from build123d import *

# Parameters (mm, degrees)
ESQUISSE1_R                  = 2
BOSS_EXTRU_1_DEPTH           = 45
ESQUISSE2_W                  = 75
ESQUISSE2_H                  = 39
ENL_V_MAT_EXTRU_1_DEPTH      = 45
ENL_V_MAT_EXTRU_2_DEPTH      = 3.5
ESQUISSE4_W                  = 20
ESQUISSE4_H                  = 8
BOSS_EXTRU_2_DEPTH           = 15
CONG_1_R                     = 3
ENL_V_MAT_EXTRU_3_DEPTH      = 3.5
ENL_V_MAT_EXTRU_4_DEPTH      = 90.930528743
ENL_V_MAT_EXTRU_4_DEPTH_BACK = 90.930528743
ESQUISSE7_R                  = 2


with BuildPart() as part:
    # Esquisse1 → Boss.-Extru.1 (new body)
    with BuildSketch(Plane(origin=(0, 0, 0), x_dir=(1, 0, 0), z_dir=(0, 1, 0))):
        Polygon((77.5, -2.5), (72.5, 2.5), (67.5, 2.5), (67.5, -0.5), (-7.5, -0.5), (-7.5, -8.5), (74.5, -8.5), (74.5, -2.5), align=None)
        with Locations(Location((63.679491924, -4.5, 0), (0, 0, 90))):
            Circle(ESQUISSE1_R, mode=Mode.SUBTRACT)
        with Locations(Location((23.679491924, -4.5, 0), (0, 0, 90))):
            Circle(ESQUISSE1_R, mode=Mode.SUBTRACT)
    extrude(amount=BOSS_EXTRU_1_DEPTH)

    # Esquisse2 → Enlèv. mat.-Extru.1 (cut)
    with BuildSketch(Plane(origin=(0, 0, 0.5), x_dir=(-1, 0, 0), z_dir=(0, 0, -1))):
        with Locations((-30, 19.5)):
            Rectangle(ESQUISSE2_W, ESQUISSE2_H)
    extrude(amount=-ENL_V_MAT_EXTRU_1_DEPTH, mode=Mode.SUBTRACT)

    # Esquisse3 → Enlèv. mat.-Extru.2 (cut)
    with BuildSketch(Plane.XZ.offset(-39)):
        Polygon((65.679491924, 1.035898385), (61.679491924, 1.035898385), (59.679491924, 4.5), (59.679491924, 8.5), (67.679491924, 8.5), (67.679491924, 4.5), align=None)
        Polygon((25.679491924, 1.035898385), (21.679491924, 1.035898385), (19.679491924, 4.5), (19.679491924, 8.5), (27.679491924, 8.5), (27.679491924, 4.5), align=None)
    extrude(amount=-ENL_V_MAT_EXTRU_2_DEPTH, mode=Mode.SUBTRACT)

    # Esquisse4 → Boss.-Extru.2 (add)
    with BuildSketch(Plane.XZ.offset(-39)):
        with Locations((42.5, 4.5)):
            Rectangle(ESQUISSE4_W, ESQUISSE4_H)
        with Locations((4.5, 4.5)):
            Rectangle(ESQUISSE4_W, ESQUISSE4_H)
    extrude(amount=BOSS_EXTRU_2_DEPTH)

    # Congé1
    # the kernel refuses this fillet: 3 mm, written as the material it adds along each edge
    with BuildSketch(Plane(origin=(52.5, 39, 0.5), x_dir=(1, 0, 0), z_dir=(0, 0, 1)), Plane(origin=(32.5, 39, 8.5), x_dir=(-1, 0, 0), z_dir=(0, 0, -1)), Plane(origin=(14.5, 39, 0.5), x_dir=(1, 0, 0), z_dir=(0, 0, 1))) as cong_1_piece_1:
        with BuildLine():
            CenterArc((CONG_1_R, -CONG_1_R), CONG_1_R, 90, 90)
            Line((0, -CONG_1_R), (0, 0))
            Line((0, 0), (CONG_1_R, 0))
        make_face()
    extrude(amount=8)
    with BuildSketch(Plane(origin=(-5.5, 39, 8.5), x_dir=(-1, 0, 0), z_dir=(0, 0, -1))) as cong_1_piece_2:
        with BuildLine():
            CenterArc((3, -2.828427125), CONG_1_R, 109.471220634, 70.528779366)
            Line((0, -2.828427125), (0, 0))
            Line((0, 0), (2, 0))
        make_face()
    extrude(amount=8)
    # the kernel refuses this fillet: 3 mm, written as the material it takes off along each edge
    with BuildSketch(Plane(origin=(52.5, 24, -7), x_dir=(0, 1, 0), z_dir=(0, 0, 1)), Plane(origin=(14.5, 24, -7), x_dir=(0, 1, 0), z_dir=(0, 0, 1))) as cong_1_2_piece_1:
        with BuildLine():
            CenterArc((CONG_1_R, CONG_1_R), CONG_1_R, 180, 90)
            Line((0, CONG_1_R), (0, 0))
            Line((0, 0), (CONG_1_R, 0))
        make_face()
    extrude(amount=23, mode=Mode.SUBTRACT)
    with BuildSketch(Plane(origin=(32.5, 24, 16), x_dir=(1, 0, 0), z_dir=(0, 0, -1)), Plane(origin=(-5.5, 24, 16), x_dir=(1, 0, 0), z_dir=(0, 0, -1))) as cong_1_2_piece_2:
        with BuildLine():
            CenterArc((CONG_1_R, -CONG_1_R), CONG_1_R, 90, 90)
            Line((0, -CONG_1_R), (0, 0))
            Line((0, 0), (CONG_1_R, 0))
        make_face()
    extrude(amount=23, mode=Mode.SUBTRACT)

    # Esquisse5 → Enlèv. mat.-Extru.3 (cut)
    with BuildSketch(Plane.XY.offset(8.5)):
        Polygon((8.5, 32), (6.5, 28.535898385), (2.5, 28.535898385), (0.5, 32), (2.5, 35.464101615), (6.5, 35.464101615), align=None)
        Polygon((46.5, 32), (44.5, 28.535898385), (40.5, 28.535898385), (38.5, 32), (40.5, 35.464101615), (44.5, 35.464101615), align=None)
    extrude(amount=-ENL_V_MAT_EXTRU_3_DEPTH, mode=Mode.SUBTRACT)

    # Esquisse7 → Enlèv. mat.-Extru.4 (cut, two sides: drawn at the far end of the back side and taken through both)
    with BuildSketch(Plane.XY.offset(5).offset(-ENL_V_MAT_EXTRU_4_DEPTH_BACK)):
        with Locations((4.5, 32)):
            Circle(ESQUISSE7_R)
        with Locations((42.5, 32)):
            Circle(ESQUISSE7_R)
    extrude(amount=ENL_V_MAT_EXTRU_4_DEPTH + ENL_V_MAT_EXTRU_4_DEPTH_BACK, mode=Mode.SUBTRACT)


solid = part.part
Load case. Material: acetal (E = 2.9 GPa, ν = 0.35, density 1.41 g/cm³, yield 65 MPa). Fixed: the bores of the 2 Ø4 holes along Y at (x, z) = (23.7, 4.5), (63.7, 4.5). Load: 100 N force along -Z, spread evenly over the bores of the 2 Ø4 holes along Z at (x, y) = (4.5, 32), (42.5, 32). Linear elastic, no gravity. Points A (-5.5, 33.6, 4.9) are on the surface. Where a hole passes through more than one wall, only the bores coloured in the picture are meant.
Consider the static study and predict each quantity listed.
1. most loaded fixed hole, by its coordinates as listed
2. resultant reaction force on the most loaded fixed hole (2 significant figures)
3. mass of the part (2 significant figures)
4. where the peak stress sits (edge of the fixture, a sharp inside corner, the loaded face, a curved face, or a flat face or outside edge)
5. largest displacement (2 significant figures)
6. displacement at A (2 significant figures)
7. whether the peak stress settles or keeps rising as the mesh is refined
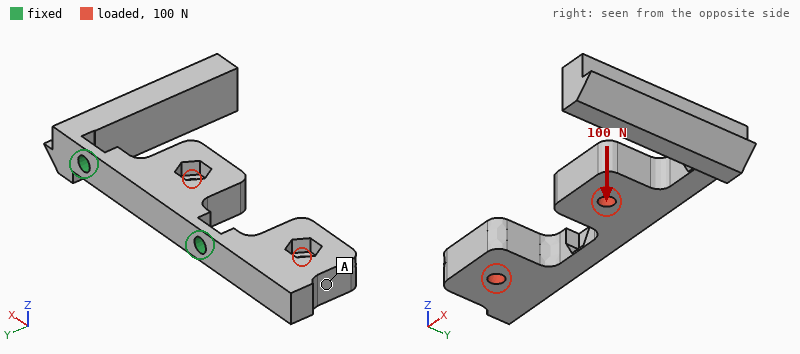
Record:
(23.7, 4.5)
81 N
16 g
edge of the fixture
1.1 mm
0.81 mm
keeps rising
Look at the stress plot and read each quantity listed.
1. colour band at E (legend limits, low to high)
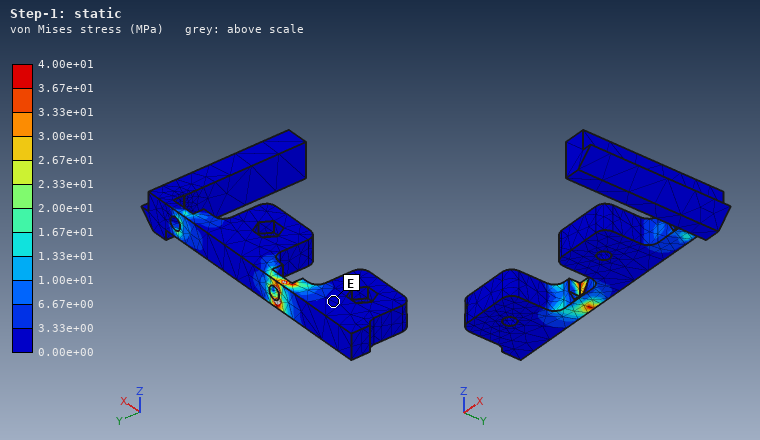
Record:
0.00e+00 to 3.33e+00 MPa
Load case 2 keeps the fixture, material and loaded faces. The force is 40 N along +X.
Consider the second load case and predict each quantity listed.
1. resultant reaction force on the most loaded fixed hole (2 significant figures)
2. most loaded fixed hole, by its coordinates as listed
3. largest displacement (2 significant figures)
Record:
24 N
(23.7, 4.5)
0.53 mm
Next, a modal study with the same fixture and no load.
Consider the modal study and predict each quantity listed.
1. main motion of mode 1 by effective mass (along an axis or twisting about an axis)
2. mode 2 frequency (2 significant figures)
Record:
along X
420 Hz
